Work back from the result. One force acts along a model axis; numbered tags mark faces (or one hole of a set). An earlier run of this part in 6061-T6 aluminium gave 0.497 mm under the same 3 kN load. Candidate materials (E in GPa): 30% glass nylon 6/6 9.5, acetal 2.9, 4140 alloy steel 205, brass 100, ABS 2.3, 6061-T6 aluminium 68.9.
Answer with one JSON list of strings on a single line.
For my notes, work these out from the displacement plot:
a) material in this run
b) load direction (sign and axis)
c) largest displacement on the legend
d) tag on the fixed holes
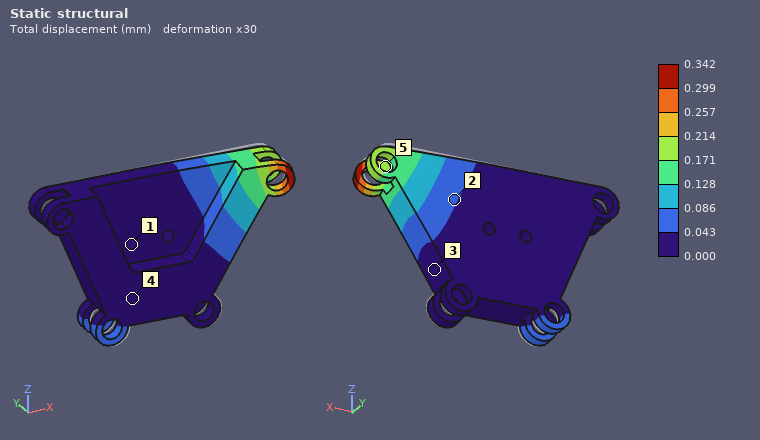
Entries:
["brass", "-Y", "0.342 mm", "1"]
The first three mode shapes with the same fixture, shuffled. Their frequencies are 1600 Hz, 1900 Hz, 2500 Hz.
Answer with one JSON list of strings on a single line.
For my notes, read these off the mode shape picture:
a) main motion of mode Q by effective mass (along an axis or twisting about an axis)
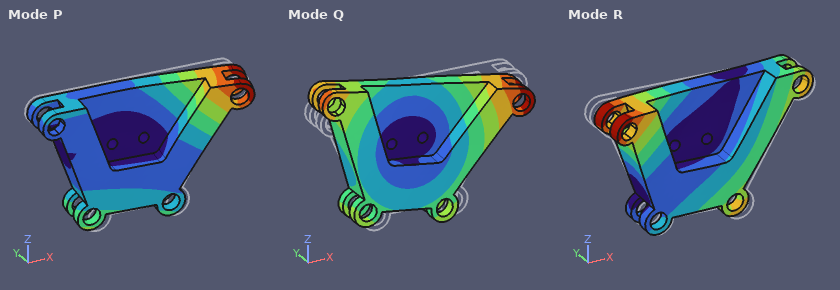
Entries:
["twisting about Y"]
